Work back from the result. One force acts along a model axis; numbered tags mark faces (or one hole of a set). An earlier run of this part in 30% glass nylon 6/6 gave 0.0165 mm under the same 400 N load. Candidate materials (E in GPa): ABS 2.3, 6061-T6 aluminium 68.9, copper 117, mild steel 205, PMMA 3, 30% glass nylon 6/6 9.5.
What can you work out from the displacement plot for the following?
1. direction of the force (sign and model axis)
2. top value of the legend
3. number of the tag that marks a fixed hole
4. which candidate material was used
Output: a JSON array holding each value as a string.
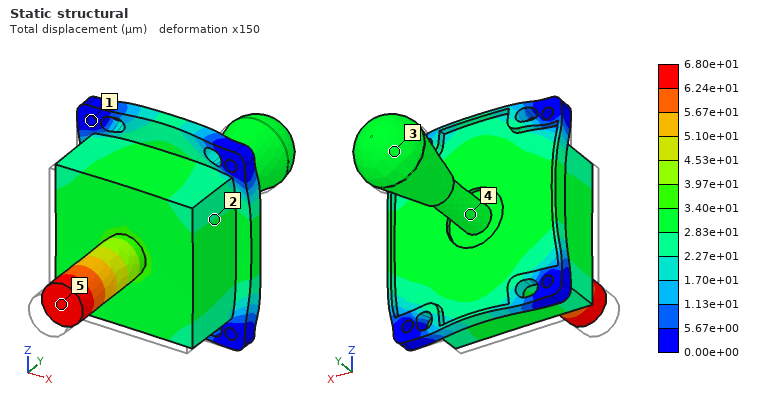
["+Y", "6.80e+01 µm", "1", "ABS"]
